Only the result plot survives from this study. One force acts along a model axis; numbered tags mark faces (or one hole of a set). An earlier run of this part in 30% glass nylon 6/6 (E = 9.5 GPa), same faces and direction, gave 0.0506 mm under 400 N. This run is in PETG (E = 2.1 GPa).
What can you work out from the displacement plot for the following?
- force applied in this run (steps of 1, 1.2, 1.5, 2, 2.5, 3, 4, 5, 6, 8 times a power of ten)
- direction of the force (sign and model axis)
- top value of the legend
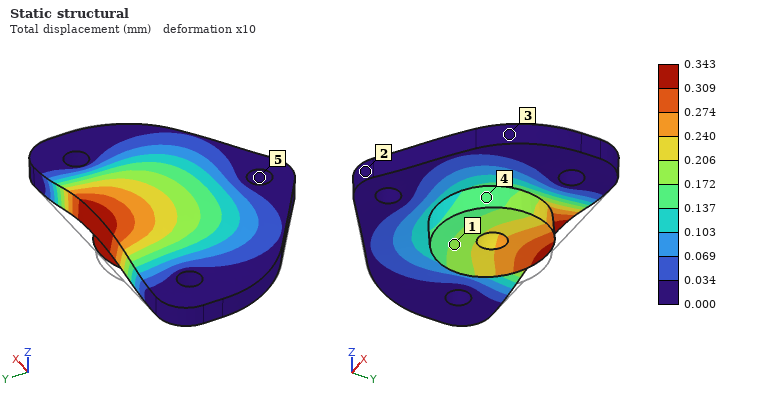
600 N
+Z
0.343 mm
